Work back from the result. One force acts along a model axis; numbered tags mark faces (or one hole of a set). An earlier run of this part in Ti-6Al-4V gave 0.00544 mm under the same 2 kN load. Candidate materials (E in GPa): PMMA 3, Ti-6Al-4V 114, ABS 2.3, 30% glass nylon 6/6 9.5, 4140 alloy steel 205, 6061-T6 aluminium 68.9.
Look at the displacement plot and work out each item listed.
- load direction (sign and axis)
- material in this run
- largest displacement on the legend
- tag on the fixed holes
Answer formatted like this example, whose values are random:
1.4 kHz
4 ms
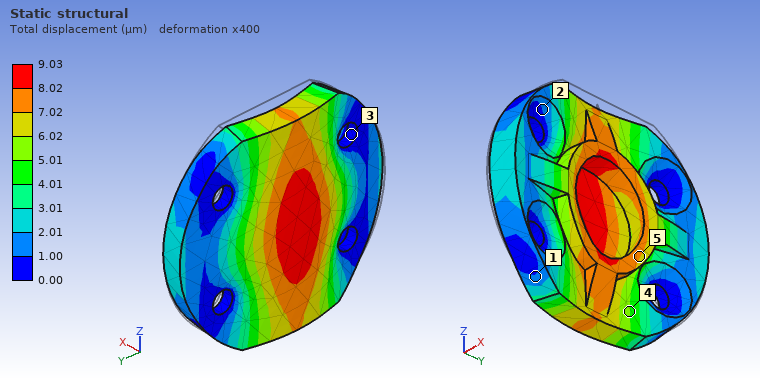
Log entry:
-X
6061-T6 aluminium
9.03 µm
3
